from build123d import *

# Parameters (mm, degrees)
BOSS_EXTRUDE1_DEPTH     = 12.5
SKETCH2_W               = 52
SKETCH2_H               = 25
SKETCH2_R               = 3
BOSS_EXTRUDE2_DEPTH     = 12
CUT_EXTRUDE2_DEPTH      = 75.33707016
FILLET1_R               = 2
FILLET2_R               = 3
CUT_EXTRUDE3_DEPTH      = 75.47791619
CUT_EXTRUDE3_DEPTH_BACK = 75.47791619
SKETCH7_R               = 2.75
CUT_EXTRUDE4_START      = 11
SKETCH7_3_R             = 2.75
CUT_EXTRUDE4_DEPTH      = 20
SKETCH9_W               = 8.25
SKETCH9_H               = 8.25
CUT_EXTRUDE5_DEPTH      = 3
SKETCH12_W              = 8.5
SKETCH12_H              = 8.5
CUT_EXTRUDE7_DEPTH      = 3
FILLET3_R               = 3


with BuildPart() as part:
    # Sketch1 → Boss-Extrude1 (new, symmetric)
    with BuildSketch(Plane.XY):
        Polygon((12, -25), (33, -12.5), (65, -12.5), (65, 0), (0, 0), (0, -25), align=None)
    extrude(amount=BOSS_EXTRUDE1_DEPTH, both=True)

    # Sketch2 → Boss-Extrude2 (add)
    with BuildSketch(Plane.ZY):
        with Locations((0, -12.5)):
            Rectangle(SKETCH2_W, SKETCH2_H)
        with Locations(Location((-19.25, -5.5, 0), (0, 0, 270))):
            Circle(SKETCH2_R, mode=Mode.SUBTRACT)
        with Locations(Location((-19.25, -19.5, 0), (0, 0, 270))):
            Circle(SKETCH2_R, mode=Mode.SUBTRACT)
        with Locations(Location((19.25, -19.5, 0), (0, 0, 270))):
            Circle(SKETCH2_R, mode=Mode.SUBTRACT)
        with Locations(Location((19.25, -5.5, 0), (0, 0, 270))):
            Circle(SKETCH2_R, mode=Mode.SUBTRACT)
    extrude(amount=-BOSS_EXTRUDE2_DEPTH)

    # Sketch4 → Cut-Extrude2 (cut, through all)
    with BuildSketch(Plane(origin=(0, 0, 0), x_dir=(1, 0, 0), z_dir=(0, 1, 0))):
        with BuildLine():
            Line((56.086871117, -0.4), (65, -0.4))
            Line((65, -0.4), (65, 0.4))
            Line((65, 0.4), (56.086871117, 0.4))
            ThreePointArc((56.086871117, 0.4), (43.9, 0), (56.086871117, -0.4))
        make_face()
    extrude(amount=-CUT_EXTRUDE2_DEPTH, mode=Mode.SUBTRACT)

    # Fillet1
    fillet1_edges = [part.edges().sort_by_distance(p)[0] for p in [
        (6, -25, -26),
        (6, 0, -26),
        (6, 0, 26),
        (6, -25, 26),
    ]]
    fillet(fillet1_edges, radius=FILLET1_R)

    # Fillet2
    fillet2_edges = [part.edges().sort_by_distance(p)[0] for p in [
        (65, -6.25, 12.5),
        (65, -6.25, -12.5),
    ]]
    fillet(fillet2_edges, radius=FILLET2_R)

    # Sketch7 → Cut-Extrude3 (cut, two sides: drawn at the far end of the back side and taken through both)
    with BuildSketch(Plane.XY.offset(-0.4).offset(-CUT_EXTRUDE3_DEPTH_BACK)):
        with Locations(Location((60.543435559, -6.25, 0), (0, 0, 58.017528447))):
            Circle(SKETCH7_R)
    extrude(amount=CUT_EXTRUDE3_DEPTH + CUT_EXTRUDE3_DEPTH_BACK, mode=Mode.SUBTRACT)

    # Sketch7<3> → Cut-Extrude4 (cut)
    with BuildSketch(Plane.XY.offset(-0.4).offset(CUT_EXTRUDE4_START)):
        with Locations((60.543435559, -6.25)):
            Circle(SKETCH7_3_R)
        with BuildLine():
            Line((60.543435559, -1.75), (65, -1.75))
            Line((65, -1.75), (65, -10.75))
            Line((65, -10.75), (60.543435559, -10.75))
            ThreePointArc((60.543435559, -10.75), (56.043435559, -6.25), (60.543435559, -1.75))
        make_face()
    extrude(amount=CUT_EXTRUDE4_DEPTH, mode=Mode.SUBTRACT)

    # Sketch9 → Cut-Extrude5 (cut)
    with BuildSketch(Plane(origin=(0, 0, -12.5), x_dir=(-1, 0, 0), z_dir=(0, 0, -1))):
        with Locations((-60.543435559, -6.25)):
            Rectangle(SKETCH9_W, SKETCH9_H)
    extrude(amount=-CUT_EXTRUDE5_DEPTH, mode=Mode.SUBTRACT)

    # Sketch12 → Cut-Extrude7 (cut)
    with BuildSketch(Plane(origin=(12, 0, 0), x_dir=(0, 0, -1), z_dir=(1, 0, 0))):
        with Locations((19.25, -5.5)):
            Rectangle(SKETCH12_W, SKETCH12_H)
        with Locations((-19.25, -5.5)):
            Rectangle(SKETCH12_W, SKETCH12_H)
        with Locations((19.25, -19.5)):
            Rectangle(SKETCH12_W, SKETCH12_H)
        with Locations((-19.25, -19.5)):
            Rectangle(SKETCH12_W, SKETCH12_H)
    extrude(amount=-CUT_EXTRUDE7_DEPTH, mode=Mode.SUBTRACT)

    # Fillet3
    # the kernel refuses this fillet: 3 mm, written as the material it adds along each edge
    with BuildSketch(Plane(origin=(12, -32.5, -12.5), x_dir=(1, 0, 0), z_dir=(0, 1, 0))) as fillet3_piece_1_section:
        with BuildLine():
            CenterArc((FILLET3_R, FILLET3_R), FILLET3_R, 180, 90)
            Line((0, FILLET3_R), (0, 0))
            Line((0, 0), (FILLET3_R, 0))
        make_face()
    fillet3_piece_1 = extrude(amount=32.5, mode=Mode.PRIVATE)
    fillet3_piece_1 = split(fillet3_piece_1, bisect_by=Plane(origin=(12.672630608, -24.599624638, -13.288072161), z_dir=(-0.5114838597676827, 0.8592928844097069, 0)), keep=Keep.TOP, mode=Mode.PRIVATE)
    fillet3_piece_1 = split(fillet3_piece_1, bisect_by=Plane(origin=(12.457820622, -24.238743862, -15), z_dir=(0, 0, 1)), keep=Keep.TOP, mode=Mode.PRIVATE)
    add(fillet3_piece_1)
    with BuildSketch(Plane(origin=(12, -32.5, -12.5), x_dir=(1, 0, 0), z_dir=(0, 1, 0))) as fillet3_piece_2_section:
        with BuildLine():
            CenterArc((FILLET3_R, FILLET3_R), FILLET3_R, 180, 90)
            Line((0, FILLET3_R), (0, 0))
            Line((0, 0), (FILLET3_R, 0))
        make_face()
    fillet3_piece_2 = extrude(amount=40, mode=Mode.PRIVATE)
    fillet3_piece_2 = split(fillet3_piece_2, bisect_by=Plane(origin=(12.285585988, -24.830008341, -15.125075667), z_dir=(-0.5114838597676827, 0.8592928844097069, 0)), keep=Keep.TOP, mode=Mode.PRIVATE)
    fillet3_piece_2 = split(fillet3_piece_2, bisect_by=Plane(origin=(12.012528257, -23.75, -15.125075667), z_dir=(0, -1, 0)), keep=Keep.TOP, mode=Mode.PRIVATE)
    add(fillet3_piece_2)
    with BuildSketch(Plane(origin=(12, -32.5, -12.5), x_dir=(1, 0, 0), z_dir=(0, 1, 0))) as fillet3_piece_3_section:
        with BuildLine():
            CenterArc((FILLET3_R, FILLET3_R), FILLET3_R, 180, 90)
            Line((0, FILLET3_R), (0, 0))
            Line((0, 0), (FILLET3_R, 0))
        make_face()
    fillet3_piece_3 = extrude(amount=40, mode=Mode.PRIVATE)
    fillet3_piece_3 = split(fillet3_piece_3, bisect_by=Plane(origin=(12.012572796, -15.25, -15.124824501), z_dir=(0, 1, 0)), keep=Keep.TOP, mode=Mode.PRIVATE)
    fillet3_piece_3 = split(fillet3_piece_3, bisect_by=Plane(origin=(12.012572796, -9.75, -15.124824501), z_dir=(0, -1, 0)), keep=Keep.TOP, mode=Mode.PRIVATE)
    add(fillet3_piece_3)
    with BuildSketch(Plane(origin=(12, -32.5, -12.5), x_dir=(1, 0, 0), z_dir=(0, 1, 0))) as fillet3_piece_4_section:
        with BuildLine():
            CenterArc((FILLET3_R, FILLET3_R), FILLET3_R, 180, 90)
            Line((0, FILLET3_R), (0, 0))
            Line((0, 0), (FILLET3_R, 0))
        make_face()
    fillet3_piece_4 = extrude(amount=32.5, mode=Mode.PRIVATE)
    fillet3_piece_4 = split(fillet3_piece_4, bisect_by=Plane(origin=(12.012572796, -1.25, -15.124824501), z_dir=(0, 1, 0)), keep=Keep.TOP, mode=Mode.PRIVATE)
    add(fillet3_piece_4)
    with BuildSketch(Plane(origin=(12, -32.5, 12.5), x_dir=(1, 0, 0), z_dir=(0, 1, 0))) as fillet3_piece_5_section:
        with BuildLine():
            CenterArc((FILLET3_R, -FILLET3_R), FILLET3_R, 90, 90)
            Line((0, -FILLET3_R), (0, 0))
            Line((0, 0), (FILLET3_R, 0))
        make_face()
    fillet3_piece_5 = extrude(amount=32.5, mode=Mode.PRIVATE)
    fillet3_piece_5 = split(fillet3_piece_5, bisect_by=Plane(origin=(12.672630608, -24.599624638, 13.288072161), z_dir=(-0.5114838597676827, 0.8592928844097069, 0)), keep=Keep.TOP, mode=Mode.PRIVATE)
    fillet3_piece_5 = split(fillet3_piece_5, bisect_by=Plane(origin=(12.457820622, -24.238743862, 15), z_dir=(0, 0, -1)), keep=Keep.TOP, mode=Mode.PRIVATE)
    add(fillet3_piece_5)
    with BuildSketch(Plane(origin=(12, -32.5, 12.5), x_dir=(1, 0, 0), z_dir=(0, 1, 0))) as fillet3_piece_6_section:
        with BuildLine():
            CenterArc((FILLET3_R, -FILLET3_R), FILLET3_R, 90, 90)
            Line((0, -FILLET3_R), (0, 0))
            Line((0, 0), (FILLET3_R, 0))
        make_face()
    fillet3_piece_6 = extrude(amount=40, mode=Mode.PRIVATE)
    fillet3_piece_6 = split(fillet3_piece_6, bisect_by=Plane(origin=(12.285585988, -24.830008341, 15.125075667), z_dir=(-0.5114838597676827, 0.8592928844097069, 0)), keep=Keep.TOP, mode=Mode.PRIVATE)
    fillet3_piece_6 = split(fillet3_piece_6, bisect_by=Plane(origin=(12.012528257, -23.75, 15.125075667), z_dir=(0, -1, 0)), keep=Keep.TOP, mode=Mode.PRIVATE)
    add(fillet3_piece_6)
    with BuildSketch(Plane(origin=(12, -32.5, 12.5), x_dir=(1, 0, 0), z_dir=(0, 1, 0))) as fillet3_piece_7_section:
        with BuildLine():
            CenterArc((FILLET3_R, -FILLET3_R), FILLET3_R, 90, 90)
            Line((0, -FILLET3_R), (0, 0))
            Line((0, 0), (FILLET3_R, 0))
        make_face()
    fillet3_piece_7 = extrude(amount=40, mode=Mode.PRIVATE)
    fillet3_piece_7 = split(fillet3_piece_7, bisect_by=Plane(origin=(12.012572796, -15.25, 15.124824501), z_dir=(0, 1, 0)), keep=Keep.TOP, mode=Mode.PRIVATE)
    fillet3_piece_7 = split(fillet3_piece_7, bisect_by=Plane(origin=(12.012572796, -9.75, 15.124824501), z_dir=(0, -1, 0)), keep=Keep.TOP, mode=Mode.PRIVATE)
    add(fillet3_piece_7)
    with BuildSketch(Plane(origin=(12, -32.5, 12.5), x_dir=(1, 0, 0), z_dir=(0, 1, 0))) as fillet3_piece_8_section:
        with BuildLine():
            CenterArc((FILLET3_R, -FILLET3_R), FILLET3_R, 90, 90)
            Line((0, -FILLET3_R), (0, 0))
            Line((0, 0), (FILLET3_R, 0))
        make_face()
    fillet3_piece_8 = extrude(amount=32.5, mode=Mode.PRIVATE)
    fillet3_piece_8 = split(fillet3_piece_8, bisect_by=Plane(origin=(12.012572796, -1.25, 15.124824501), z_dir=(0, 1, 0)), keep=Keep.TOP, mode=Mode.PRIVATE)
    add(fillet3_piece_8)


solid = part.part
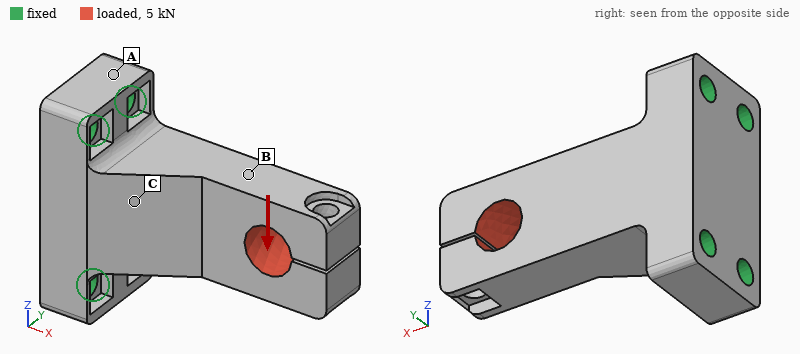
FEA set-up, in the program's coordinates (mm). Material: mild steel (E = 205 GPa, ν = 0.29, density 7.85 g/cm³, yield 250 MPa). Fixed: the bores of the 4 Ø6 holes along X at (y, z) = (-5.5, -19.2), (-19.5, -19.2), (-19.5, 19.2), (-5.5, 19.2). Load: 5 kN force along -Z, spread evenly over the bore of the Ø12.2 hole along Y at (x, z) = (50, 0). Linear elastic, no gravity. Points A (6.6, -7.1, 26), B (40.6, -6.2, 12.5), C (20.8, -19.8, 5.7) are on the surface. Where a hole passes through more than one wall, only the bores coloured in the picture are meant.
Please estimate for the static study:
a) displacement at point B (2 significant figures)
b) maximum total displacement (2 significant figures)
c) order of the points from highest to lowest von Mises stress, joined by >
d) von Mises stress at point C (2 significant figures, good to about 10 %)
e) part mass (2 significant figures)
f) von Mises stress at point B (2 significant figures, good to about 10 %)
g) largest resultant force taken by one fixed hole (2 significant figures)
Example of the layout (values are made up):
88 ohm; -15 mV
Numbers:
30 µm; 79 µm; B > C > A; 38 MPa; 250 g; 71 MPa; 4.0 kN
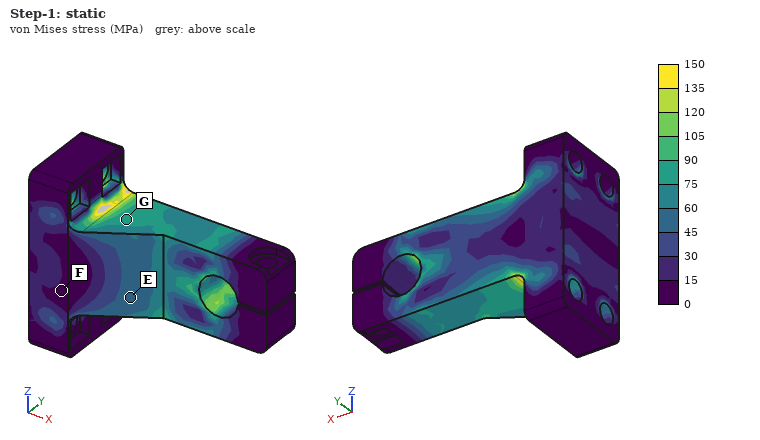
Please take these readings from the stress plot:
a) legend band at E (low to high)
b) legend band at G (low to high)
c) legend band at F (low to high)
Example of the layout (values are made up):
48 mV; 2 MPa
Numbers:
45 to 60 MPa; 75 to 90 MPa; 0 to 15 MPa
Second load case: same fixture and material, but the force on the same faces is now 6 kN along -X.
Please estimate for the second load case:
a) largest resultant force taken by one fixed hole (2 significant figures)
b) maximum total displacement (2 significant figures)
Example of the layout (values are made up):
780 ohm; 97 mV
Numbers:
2.7 kN; 36 µm
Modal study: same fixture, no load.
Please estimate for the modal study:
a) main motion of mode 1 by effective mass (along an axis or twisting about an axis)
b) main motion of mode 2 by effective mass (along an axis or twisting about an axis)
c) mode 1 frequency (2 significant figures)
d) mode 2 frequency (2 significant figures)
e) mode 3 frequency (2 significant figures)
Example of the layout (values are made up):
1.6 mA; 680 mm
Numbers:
along Y; along Z; 4600 Hz; 6200 Hz; 8800 Hz
